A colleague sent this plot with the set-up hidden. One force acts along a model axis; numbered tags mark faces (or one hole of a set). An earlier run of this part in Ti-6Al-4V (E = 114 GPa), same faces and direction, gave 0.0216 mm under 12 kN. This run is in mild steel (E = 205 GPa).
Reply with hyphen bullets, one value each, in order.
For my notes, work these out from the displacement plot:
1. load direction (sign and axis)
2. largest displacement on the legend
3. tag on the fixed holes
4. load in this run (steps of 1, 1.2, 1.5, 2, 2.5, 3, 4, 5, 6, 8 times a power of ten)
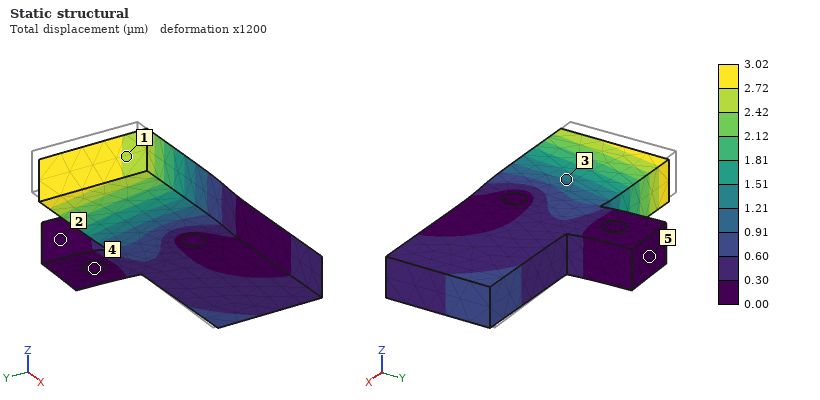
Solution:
- +X
- 3.02 µm
- 4
- 3 kN
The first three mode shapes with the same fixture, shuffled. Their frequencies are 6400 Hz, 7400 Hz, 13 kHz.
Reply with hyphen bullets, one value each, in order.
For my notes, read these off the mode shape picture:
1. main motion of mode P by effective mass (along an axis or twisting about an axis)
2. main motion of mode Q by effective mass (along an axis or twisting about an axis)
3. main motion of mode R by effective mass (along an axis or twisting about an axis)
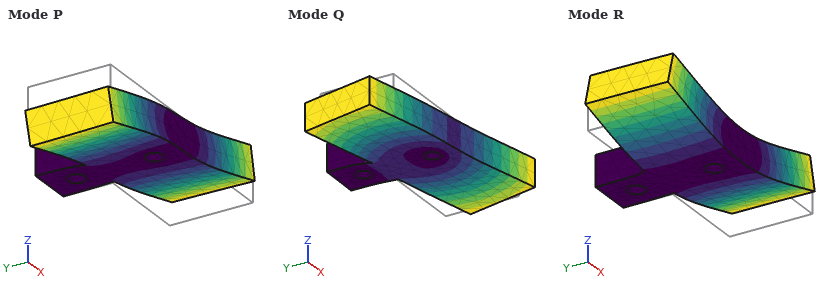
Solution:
- twisting about Y
- twisting about Z
- along Z
